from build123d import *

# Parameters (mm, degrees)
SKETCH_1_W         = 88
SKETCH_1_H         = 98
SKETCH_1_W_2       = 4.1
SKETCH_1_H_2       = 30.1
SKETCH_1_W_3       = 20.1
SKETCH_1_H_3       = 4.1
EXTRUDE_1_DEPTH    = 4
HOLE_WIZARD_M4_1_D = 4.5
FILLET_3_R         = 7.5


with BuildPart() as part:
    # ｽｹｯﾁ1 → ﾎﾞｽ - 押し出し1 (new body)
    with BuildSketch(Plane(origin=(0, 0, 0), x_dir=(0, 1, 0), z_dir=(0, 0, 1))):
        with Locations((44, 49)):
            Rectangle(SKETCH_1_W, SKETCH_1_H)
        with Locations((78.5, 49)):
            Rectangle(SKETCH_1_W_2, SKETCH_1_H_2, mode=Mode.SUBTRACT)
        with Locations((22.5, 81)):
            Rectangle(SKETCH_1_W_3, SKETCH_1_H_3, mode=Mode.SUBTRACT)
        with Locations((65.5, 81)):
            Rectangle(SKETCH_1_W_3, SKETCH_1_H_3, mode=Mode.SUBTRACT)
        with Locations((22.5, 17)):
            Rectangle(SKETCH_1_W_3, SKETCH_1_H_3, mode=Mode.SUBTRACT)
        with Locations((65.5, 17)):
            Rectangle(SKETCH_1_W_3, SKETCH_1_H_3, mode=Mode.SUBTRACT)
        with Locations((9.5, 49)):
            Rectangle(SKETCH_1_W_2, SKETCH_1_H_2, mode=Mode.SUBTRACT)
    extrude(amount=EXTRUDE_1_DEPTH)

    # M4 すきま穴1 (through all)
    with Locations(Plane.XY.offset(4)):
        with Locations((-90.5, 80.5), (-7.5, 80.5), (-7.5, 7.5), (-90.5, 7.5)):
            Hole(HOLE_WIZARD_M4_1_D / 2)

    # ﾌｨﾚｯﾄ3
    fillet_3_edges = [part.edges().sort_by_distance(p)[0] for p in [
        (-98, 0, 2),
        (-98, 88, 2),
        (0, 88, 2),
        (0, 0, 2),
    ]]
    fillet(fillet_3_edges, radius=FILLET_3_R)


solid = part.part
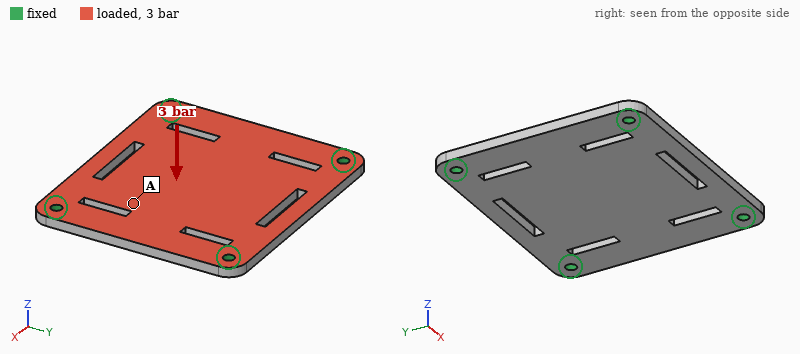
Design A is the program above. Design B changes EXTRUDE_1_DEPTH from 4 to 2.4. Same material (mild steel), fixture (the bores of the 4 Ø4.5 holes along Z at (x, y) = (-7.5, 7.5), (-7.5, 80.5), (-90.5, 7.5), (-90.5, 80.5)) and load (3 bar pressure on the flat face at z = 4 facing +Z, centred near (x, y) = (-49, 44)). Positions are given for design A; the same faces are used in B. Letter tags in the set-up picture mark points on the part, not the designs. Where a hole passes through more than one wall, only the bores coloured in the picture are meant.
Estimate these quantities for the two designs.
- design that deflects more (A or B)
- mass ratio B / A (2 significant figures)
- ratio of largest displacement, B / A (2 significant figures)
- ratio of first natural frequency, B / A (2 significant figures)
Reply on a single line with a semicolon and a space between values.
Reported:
B; 0.60; 4.3; 0.62
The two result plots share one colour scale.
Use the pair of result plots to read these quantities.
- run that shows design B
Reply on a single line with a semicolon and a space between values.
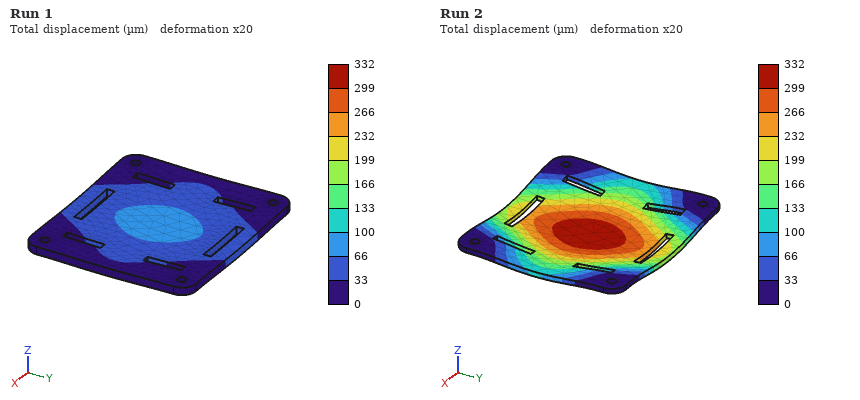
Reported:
Run 2
